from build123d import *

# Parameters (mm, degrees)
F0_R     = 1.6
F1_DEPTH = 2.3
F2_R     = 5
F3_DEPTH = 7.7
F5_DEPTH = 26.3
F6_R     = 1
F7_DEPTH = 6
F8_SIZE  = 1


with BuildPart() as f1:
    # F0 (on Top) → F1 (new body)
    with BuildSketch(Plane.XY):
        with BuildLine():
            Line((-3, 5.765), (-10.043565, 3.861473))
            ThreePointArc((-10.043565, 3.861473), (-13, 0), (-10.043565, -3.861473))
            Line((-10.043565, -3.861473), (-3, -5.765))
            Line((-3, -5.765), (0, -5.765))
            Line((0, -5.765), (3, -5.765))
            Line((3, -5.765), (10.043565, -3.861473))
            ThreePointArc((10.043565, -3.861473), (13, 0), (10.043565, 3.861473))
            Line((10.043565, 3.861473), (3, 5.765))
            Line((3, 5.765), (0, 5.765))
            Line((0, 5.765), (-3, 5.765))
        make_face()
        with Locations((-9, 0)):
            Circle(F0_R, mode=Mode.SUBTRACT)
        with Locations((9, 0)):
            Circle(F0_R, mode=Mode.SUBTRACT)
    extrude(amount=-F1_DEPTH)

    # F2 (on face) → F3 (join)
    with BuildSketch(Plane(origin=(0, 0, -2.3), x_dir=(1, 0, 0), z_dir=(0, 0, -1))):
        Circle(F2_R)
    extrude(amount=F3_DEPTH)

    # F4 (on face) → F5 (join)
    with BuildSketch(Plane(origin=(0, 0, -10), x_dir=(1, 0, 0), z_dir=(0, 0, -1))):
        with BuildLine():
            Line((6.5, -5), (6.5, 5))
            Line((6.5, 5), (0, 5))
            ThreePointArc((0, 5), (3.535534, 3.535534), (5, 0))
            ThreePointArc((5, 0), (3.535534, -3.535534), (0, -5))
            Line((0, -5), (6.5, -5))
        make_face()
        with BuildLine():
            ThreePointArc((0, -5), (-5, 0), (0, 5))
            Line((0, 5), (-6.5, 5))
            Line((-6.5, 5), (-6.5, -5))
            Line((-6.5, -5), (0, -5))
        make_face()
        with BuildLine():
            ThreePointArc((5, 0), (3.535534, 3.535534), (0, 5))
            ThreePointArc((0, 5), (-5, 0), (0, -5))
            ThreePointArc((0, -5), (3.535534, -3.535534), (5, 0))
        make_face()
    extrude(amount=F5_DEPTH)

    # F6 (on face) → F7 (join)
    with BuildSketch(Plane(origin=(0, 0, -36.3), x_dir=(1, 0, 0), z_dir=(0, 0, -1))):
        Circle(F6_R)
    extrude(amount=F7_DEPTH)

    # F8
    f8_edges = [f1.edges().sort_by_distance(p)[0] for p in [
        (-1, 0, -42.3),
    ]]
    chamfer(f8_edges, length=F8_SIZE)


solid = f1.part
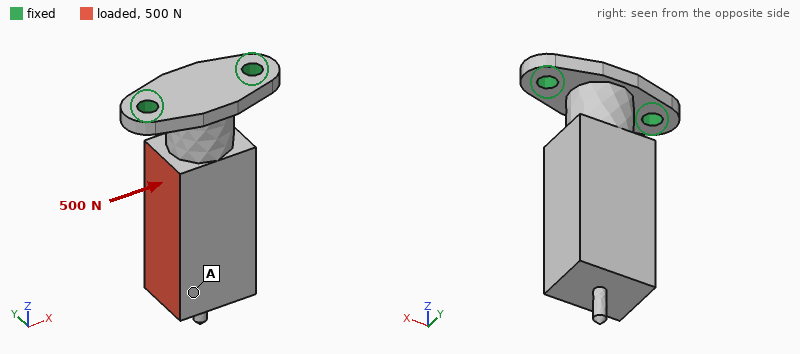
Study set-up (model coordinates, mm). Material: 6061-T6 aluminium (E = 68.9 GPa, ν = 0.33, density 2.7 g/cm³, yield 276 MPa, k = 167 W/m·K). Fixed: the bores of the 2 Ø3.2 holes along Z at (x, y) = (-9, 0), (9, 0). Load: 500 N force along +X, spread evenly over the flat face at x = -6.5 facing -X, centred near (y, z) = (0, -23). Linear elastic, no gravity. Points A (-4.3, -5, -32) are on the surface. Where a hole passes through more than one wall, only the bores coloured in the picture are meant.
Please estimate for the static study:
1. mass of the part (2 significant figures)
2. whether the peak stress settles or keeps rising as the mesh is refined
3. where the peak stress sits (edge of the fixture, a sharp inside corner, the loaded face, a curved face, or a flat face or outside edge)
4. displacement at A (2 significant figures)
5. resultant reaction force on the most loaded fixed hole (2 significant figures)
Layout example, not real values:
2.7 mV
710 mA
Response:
12 g
keeps rising
edge of the fixture
0.15 mm
880 N
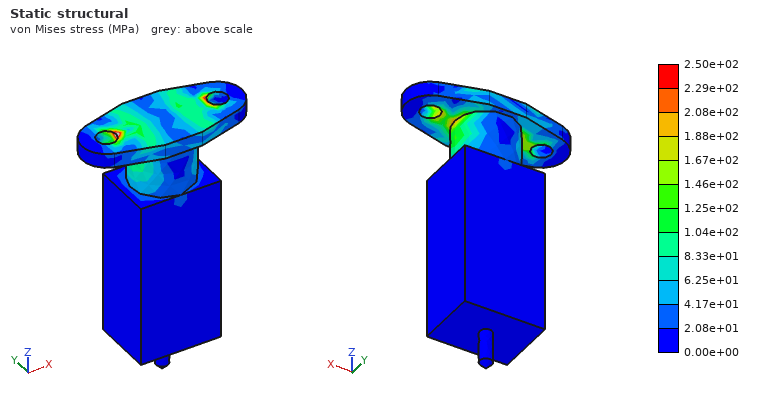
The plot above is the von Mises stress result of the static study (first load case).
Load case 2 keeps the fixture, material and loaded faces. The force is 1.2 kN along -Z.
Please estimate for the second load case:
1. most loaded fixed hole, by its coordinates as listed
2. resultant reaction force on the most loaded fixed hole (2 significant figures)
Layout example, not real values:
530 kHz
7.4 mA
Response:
(-9, 0)
1.2 kN
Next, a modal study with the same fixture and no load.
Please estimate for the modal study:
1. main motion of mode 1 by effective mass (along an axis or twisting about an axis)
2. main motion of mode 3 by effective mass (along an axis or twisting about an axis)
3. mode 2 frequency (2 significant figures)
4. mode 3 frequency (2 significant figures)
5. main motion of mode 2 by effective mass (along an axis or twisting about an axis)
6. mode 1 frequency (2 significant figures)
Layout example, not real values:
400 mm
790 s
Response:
along Y
along Z
3300 Hz
13 kHz
along X
1600 Hz
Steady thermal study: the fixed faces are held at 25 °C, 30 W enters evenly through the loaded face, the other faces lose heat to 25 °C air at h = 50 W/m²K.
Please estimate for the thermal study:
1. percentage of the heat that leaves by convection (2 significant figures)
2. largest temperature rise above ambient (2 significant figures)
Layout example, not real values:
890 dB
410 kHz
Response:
11 %
56 K
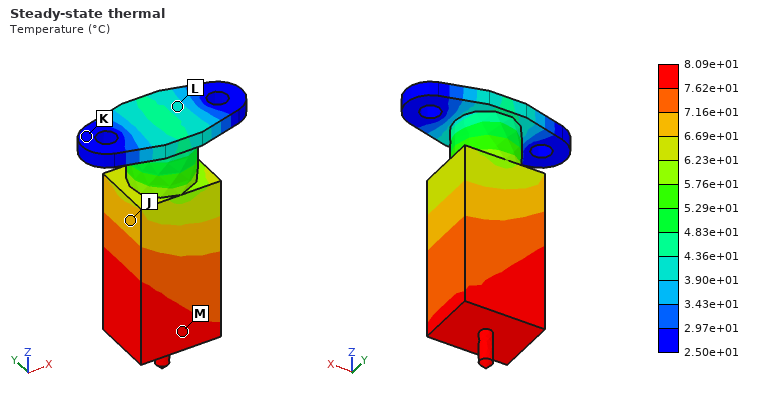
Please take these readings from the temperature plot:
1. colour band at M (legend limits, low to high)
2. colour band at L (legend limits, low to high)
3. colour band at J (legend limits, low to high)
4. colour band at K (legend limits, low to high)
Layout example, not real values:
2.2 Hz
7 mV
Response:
7.62e+01 to 8.09e+01 °C
3.90e+01 to 4.36e+01 °C
6.69e+01 to 7.16e+01 °C
2.50e+01 to 2.97e+01 °C
